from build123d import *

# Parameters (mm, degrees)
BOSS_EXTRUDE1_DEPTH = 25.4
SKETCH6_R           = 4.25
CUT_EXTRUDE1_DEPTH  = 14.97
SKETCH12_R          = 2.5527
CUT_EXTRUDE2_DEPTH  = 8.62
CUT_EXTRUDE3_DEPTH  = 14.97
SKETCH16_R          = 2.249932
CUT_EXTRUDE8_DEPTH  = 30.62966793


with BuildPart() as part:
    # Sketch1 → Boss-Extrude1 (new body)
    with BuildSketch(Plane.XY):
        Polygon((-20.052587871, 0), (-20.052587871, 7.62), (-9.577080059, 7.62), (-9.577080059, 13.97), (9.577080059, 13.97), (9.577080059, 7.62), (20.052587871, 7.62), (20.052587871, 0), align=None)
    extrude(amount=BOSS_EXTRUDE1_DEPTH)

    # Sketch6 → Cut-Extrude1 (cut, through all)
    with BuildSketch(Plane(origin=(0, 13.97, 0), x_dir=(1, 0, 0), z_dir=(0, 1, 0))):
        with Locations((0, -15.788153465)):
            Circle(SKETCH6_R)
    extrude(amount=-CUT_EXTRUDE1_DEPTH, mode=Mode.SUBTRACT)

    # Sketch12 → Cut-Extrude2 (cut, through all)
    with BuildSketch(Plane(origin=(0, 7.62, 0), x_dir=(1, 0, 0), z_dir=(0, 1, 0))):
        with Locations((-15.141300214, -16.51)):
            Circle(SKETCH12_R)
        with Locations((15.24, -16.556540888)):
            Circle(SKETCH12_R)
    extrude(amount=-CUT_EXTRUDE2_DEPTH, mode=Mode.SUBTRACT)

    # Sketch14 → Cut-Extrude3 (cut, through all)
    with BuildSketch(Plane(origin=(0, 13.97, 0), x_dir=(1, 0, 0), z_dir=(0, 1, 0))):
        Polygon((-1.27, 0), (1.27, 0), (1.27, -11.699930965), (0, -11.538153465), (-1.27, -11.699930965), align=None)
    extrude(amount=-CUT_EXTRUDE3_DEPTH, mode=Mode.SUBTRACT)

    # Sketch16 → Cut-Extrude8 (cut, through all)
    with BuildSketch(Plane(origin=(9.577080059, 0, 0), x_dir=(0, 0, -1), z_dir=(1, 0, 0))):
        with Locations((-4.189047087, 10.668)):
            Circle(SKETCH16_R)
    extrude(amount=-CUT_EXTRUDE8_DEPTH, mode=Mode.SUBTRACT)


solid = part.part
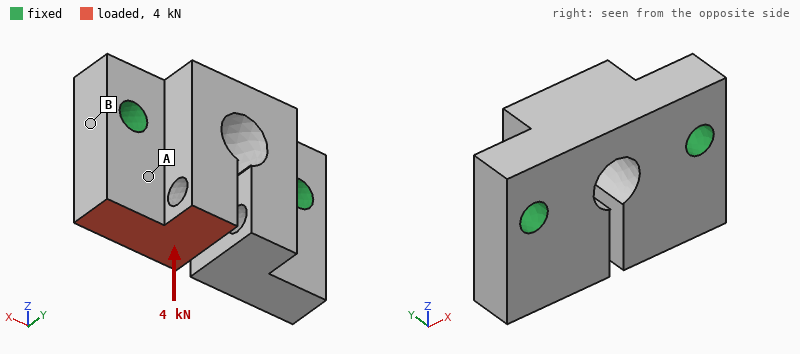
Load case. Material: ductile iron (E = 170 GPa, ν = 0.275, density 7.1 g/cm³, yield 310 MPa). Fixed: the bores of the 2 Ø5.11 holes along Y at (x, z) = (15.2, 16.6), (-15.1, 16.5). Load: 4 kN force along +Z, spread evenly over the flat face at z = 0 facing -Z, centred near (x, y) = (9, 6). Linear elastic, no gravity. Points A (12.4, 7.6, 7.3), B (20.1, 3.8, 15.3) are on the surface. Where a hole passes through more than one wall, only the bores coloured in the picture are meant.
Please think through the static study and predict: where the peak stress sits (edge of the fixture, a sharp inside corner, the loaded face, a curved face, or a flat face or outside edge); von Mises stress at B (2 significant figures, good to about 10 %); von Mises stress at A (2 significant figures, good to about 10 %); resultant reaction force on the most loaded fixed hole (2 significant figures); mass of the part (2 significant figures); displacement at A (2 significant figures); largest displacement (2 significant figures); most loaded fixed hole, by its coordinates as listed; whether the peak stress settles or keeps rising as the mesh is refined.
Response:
edge of the fixture
16 MPa
35 MPa
3.5 kN
64 g
4.5 µm
14 µm
(15.2, 16.6)
keeps rising
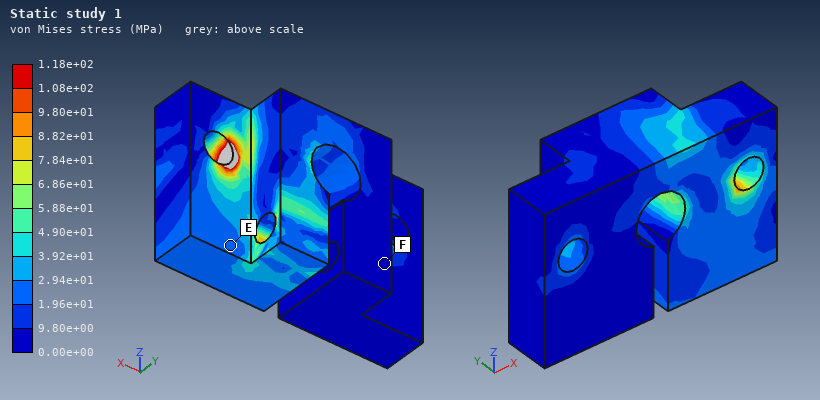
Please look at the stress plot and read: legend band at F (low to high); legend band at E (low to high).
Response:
0.00e+00 to 9.80e+00 MPa
1.96e+01 to 2.94e+01 MPa
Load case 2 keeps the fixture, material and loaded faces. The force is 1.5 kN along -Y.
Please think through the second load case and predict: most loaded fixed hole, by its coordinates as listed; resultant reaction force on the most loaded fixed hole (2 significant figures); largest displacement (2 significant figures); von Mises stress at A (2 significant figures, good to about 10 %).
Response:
(15.2, 16.6)
1.5 kN
26 µm
38 MPa
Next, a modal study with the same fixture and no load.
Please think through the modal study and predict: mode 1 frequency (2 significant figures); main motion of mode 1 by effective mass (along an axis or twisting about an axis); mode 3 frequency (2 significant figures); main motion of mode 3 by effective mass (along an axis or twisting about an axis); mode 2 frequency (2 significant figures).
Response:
14 kHz
along Y
16 kHz
along Z
15 kHz
